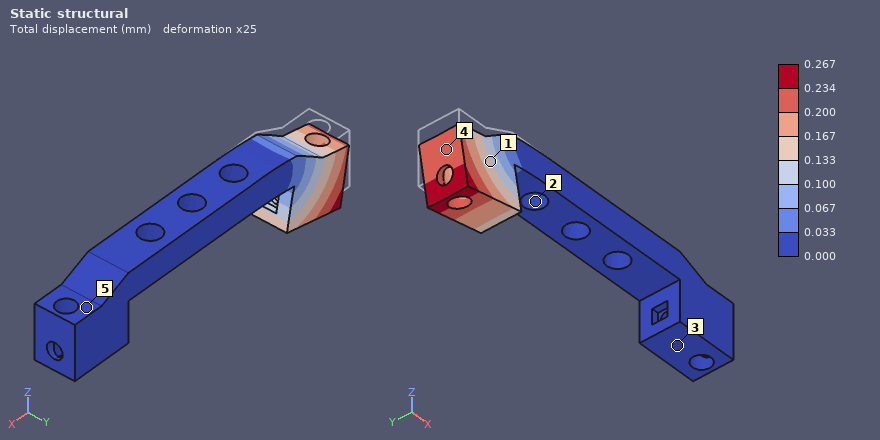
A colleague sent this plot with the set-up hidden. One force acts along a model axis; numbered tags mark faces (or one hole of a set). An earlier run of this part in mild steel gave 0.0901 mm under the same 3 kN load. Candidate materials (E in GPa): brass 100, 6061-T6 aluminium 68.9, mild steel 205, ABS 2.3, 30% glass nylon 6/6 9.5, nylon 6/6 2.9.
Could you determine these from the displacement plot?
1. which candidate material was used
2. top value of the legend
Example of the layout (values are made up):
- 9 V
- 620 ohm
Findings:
- 6061-T6 aluminium
- 0.267 mm
